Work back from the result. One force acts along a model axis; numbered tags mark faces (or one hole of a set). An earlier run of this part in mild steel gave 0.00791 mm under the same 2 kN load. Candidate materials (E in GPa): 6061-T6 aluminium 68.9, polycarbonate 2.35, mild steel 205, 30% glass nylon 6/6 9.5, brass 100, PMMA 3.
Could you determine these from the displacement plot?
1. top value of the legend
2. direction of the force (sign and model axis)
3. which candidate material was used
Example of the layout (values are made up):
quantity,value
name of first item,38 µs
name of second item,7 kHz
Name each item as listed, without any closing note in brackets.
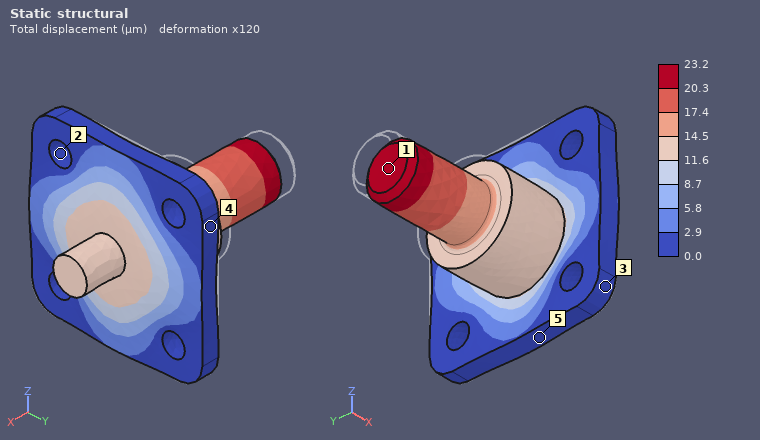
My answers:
quantity,value
top value of the legend,23.2 µm
direction of the force,+X
which candidate material was used,6061-T6 aluminium
